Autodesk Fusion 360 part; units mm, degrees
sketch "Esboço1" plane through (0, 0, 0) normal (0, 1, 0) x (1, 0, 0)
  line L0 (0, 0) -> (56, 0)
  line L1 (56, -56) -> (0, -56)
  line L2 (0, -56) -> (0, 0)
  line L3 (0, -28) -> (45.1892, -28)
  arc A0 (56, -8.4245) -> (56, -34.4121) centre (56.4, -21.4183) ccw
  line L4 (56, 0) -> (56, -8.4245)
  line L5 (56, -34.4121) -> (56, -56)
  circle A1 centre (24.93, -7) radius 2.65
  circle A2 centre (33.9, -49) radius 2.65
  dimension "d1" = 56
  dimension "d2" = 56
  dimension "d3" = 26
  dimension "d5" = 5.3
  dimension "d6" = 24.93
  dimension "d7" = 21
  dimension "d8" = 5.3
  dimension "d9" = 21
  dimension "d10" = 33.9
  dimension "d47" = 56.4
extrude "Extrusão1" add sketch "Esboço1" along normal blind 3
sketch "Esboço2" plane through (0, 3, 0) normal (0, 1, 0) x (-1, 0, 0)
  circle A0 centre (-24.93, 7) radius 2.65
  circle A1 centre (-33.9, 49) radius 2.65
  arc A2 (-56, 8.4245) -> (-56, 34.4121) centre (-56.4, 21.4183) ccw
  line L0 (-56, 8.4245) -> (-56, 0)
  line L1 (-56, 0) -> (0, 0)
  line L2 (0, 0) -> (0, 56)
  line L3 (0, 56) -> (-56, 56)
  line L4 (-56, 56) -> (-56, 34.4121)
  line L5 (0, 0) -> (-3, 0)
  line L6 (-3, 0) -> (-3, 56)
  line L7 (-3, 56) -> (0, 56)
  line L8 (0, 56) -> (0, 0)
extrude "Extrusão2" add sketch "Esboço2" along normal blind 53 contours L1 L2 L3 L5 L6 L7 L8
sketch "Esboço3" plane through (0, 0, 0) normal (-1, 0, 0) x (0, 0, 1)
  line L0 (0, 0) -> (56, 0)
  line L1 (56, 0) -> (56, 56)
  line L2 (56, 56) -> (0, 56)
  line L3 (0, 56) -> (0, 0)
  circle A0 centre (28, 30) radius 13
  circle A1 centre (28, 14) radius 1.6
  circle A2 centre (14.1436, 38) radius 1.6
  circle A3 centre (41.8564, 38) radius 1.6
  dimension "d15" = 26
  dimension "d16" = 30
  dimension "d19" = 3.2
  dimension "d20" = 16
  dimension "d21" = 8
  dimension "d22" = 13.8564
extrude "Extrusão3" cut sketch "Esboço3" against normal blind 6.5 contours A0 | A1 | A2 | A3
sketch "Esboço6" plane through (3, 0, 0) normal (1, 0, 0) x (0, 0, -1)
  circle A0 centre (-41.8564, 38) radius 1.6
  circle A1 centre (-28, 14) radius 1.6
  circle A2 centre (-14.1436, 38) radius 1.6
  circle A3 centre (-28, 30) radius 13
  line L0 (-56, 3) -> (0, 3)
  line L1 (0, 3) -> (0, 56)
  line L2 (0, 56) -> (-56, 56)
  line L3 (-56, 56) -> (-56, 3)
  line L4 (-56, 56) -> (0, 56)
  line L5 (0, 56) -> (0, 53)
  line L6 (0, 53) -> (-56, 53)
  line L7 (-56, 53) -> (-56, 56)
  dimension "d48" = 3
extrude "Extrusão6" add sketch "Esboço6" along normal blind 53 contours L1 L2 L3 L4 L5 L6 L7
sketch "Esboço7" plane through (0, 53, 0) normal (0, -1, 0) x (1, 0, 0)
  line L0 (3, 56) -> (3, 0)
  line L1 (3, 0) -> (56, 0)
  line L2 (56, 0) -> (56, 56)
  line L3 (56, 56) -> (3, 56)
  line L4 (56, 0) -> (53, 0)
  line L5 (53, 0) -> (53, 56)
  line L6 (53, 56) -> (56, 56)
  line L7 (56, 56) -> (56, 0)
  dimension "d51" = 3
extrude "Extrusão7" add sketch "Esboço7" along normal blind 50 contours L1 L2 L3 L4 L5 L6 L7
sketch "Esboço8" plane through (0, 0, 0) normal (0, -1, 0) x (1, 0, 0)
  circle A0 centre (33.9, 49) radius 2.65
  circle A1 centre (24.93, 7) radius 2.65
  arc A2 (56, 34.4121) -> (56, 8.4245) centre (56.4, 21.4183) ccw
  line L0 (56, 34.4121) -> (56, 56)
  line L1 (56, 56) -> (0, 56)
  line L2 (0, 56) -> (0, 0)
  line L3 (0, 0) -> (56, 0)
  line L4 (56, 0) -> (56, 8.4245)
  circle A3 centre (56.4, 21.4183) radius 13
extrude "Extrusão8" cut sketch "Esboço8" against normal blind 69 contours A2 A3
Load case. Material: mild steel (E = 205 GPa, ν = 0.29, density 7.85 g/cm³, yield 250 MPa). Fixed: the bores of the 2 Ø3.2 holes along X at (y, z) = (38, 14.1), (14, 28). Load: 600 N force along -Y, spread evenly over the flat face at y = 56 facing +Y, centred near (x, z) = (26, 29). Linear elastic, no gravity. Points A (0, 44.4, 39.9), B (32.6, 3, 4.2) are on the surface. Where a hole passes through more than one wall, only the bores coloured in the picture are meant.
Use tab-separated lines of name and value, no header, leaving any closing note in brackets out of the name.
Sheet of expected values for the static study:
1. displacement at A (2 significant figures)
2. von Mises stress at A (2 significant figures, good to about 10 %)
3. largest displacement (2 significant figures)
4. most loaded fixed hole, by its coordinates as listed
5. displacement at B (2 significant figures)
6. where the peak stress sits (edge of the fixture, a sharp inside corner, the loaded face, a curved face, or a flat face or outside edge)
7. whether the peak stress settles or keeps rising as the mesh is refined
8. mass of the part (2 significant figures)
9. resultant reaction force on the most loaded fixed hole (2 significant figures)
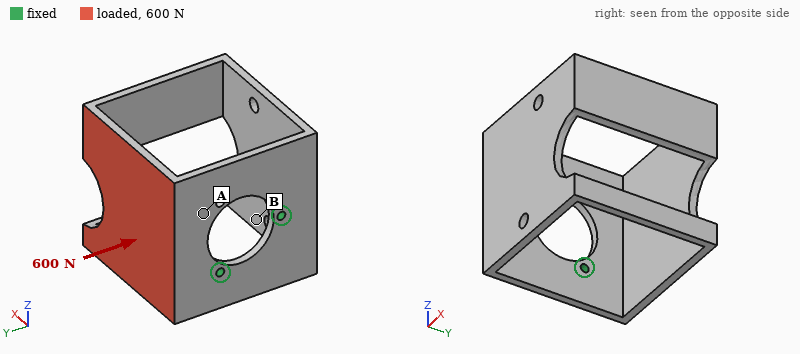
displacement at A	0.064 mm
von Mises stress at A	51 MPa
largest displacement	0.34 mm
most loaded fixed hole, by its coordinates as listed	(14, 28)
displacement at B	0.18 mm
where the peak stress sits	edge of the fixture
whether the peak stress settles or keeps rising as the mesh is refined	keeps rising
mass of the part	220 g
resultant reaction force on the most loaded fixed hole	440 N
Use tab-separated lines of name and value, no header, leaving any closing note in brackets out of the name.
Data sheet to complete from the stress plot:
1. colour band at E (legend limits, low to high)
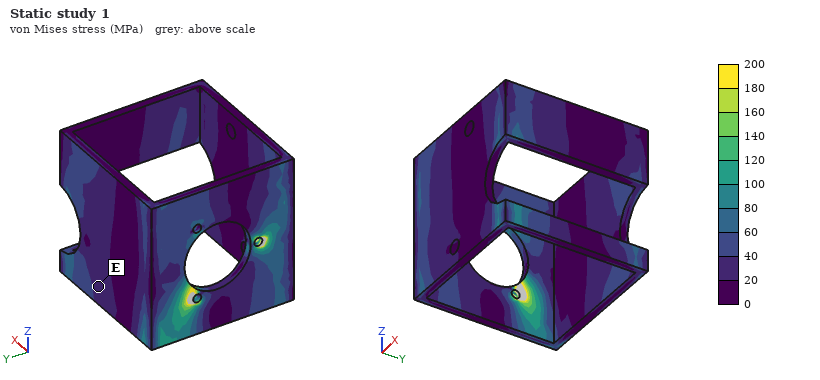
colour band at E	20 to 40 MPa
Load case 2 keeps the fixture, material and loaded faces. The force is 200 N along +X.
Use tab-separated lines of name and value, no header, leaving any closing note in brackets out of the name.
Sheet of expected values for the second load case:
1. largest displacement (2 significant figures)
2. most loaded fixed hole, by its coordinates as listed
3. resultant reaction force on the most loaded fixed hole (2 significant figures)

largest displacement	0.12 mm
most loaded fixed hole, by its coordinates as listed	(38, 14.1)
resultant reaction force on the most loaded fixed hole	210 N
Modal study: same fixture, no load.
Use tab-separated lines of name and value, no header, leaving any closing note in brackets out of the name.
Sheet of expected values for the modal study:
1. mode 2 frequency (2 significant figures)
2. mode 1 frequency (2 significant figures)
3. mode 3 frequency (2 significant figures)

mode 2 frequency	670 Hz
mode 1 frequency	460 Hz
mode 3 frequency	1300 Hz
